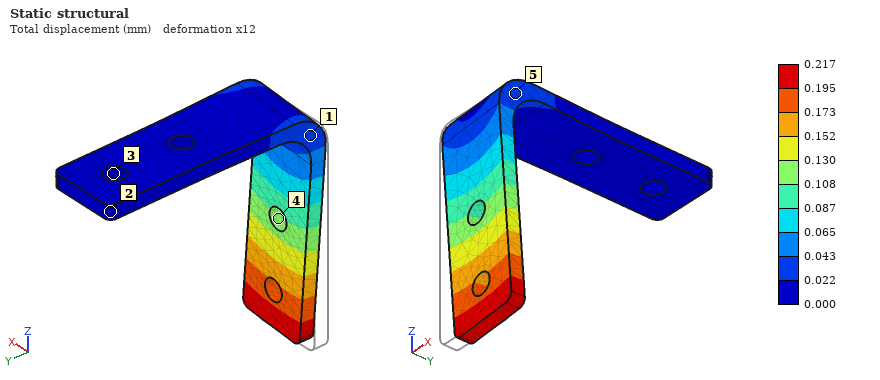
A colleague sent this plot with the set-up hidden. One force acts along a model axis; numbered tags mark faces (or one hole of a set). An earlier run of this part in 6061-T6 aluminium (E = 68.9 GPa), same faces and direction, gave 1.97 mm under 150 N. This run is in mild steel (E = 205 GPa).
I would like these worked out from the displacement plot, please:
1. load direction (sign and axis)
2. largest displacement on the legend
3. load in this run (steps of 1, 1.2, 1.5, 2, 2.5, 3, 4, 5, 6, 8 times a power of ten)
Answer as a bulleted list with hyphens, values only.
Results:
- +X
- 0.217 mm
- 50 N
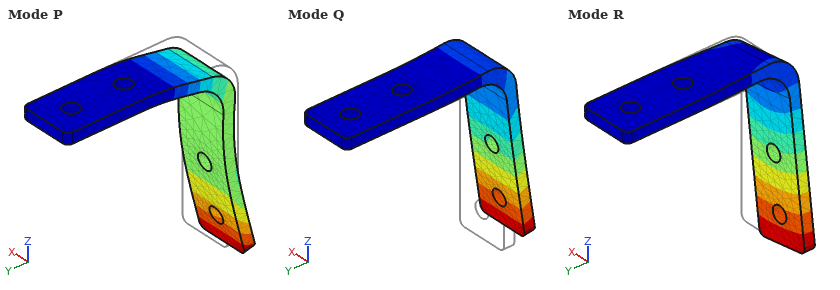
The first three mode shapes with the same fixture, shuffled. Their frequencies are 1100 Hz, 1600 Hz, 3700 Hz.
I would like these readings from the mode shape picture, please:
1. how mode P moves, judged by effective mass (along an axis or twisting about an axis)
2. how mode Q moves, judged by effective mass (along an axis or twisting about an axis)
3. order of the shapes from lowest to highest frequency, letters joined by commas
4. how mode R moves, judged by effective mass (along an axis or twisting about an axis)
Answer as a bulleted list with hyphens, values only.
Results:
- along Z
- along Y
- Q, R, P
- along X
